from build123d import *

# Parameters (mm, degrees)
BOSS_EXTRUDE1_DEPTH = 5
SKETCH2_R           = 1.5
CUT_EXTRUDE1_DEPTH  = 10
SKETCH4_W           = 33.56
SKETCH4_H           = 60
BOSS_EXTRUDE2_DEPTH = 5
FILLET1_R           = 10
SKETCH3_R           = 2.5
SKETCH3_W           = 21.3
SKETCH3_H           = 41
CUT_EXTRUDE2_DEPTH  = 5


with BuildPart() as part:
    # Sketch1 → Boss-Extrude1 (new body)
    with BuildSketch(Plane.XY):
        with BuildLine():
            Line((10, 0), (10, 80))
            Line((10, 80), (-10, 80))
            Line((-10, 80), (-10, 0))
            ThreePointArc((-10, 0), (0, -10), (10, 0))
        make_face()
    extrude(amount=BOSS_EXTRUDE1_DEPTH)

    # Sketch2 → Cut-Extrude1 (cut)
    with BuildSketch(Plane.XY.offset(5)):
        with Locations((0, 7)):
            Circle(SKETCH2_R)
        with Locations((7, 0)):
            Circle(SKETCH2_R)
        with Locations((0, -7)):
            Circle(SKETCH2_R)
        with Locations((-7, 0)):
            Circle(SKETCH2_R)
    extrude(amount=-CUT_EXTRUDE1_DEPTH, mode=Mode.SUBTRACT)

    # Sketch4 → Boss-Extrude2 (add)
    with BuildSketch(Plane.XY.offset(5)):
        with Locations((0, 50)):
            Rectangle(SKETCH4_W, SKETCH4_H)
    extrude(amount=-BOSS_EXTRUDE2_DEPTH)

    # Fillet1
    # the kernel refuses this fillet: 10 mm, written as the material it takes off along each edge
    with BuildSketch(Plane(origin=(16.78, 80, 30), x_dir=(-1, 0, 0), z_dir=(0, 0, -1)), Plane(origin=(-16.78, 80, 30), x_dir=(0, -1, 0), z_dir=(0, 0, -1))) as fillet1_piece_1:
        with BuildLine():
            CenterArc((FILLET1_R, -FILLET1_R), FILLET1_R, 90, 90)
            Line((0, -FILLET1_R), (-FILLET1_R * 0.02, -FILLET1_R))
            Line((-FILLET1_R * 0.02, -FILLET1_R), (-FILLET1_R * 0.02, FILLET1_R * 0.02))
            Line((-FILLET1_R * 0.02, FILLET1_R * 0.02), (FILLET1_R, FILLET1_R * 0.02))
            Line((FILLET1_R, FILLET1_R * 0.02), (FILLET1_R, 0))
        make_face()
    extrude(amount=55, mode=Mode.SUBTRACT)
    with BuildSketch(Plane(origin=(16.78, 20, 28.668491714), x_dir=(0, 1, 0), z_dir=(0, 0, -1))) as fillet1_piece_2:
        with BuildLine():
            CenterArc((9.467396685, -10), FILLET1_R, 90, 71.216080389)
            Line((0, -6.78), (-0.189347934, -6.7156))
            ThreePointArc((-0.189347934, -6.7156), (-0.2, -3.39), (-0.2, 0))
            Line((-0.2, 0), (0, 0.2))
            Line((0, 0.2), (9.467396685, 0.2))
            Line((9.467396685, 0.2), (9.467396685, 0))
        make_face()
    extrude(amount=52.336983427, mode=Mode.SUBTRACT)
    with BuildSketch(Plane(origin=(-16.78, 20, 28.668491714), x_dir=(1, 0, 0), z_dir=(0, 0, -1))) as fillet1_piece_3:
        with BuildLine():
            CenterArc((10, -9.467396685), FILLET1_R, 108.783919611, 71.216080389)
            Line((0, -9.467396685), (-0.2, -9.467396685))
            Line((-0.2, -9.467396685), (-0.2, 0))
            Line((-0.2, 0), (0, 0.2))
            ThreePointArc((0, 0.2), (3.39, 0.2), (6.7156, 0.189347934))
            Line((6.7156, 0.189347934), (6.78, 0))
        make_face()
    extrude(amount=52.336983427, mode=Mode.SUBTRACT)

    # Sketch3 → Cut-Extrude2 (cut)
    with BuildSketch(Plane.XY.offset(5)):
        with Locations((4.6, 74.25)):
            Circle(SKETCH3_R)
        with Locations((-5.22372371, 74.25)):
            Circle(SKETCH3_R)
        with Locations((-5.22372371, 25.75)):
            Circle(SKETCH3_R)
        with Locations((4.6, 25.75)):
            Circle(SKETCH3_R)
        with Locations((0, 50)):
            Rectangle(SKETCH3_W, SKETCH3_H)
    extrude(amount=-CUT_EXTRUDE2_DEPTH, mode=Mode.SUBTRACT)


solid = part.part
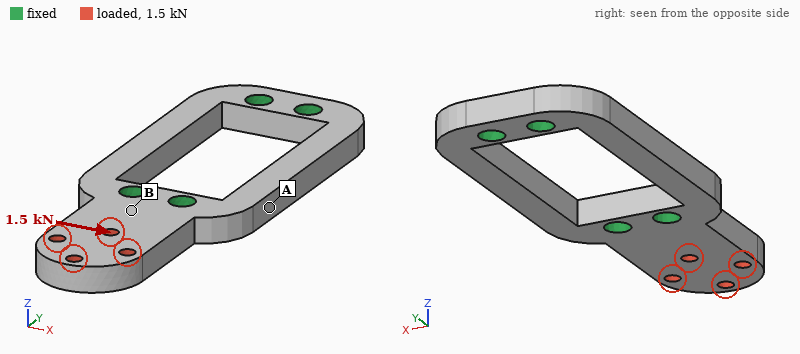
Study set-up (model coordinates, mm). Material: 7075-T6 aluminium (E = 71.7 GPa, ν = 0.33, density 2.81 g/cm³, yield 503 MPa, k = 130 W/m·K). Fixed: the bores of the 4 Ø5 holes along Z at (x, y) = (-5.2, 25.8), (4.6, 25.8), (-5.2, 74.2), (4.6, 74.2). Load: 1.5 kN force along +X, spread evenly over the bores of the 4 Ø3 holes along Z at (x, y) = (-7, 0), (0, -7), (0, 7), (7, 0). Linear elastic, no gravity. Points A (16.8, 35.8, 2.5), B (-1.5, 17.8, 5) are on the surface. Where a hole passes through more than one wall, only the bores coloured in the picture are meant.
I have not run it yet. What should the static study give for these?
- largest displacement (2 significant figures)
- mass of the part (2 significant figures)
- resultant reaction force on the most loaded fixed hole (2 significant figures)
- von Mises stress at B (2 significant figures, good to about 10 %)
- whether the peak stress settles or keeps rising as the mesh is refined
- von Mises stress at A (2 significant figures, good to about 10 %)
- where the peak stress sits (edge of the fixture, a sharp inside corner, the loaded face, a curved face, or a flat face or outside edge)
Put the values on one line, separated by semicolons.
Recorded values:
68 µm; 21 g; 2.5 kN; 41 MPa; keeps rising; 14 MPa; edge of the fixture
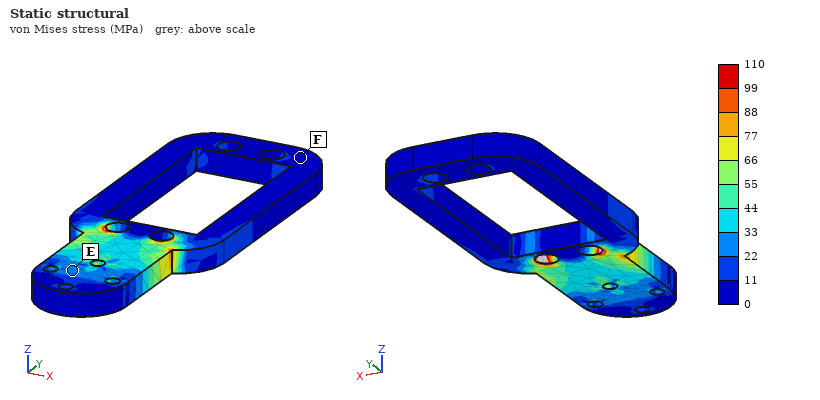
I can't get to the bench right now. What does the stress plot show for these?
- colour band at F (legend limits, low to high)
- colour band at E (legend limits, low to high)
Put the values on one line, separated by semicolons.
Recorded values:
0 to 11 MPa; 22 to 33 MPa
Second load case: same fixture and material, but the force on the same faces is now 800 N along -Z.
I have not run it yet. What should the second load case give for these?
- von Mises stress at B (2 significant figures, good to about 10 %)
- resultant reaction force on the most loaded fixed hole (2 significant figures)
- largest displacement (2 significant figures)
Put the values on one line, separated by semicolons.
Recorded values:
150 MPa; 430 N; 0.41 mm
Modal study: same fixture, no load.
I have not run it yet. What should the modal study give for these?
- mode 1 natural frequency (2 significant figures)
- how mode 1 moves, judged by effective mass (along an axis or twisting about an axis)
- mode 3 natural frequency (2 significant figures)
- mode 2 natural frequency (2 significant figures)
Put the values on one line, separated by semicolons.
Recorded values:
4100 Hz; along Z; 8700 Hz; 8400 Hz
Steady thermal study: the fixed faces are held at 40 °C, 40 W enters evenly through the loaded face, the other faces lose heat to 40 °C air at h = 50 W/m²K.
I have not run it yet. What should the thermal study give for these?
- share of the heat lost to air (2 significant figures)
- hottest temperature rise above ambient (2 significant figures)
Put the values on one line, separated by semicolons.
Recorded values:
9.1 %; 77 K
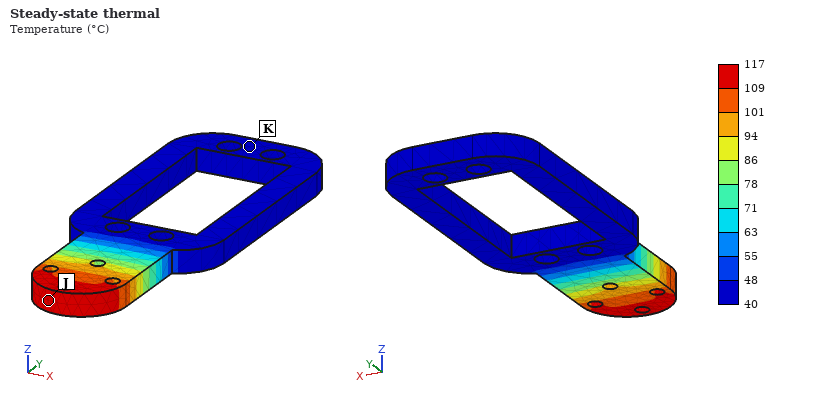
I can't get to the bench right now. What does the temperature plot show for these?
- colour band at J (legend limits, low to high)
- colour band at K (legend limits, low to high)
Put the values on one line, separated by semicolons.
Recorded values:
109 to 117 °C; 40 to 48 °C
